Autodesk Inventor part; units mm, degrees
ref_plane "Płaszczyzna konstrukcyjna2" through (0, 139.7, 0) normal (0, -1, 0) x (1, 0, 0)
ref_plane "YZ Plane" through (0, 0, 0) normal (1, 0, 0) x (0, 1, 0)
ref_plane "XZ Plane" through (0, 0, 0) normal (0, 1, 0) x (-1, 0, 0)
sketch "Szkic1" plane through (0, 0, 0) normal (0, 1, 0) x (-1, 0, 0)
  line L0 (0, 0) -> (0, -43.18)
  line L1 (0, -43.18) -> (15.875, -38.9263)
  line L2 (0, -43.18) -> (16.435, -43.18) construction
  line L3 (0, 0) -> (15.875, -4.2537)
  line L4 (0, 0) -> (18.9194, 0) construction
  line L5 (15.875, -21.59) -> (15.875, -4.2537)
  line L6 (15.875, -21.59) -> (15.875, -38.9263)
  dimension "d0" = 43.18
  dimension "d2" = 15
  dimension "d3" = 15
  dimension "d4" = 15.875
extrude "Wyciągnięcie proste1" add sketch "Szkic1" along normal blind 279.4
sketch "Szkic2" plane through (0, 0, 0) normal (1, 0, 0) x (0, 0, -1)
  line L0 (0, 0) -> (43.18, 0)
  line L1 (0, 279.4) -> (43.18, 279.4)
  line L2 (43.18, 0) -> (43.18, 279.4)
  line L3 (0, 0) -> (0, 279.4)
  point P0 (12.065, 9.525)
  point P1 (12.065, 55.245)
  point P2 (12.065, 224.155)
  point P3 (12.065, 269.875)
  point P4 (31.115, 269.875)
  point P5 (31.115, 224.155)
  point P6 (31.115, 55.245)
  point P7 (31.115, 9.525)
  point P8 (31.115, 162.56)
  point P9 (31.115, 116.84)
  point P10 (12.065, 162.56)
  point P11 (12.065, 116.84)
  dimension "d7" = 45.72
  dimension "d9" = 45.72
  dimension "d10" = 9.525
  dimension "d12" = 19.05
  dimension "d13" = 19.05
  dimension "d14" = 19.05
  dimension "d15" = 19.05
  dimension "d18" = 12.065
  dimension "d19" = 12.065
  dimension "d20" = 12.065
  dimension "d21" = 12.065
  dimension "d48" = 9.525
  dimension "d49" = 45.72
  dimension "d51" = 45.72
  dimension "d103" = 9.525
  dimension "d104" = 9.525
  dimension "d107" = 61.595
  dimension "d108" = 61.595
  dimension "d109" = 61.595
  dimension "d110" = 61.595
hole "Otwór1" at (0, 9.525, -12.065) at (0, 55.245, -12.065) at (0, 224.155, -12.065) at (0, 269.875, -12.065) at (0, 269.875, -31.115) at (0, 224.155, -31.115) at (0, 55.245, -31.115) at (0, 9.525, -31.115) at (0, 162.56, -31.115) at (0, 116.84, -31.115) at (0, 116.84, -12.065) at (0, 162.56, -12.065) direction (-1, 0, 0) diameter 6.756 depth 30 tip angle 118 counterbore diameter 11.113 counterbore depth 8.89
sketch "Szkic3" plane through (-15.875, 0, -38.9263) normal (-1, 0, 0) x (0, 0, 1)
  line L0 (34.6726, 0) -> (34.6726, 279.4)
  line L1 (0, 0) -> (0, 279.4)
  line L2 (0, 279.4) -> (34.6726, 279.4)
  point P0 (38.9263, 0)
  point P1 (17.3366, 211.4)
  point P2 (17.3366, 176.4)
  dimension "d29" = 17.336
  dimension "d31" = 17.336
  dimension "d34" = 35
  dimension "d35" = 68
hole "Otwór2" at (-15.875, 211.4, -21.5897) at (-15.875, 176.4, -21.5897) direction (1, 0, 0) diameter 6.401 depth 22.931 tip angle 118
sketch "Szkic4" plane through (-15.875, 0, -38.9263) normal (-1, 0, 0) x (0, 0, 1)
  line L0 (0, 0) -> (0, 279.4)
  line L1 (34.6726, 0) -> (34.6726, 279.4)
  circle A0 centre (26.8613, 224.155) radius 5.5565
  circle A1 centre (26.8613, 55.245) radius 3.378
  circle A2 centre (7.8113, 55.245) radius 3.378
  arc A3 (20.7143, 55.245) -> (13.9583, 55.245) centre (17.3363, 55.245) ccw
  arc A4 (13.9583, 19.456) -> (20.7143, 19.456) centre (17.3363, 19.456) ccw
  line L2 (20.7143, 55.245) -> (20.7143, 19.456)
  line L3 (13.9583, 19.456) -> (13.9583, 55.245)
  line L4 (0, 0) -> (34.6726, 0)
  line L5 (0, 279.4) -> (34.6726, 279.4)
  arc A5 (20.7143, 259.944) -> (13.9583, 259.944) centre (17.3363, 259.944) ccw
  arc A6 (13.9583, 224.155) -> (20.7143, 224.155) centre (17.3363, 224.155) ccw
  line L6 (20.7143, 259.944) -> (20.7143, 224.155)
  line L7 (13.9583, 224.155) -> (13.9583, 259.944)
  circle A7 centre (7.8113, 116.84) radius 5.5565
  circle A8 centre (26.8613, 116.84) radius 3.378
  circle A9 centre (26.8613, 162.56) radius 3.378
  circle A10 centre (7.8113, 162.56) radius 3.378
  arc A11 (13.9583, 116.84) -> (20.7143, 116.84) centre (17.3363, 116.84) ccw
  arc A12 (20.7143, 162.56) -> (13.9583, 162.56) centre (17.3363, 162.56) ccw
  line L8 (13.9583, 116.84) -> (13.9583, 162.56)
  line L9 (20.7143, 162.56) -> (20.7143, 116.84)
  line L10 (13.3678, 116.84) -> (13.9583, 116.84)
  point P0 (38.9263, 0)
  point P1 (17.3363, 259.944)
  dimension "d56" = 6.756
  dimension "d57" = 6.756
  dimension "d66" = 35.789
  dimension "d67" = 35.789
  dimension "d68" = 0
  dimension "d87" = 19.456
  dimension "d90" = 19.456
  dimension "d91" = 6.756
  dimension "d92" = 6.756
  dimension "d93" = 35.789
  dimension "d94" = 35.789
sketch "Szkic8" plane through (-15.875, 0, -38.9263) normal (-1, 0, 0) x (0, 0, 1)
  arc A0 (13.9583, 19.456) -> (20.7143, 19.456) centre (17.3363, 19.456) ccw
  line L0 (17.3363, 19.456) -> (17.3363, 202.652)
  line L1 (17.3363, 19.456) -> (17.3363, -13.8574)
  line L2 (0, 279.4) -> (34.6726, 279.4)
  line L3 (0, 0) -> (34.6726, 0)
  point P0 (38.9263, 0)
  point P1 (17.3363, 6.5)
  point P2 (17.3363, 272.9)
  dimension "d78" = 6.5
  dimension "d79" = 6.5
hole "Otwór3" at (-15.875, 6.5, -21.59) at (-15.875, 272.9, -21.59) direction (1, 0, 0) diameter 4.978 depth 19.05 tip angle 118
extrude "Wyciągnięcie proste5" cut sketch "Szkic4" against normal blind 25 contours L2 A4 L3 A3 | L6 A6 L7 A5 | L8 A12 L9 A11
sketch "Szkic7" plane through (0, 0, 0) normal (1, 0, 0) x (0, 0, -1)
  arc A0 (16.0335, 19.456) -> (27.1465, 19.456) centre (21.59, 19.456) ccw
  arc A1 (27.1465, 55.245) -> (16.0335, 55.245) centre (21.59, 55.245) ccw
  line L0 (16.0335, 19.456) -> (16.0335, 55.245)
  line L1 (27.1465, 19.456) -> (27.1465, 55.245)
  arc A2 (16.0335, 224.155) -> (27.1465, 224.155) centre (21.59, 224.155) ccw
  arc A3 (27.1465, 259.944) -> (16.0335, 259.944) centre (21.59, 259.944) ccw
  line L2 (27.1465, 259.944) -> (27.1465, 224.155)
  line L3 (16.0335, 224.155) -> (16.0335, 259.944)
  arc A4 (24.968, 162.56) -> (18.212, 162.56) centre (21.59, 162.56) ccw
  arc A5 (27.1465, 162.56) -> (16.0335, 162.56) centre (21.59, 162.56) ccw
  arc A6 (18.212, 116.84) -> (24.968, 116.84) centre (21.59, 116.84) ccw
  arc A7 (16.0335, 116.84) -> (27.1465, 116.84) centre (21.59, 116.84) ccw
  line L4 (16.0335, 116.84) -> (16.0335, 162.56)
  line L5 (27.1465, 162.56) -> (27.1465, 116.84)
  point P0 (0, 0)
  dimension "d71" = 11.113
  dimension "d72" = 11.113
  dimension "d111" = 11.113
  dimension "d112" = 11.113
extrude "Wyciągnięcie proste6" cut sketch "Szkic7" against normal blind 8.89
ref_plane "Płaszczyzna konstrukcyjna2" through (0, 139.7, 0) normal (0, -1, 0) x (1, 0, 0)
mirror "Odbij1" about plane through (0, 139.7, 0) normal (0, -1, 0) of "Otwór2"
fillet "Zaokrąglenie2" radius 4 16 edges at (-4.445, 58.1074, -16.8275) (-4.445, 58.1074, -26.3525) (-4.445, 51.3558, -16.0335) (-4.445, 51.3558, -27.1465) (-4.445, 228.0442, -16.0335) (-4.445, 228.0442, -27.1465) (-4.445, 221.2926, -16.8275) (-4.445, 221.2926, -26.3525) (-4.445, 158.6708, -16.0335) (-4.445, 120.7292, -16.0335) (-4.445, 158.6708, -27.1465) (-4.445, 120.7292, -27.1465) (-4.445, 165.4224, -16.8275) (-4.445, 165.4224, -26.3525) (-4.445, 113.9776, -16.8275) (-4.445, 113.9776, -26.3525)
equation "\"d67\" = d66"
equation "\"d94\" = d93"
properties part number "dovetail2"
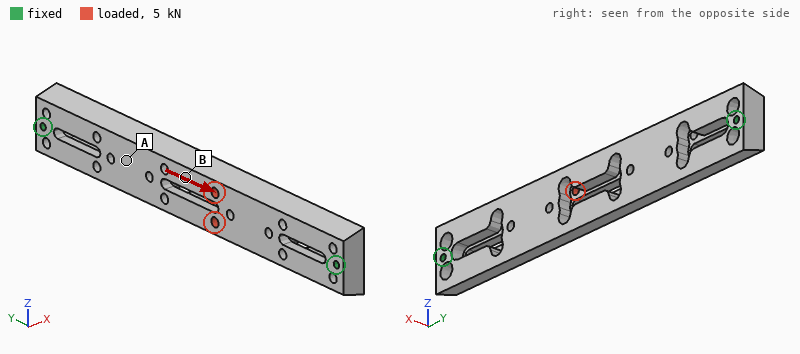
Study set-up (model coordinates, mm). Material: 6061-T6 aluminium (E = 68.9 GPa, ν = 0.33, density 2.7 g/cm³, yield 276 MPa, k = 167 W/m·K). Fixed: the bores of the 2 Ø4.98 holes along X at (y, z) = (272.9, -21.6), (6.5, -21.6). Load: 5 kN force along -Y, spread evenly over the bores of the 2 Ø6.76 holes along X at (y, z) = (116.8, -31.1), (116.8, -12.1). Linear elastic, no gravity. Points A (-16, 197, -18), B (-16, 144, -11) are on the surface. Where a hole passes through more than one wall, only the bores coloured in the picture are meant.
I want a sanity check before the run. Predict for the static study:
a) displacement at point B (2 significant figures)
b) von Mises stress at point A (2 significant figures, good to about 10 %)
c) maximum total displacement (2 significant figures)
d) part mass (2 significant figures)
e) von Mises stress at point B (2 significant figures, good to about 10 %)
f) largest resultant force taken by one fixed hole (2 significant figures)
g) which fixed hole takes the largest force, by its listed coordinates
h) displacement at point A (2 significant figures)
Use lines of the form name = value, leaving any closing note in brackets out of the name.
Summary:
displacement at point B = 30 µm
von Mises stress at point A = 5.2 MPa
maximum total displacement = 31 µm
part mass = 370 g
von Mises stress at point B = 12 MPa
largest resultant force taken by one fixed hole = 2.9 kN
which fixed hole takes the largest force, by its listed coordinates = (6.5, -21.6)
displacement at point A = 24 µm
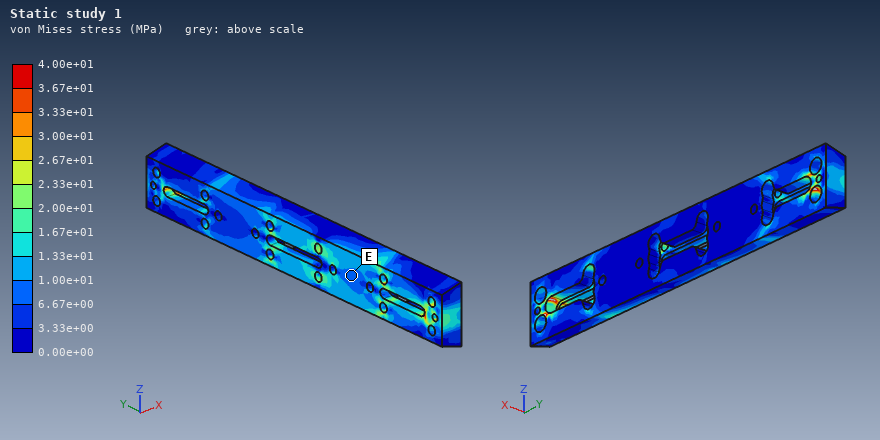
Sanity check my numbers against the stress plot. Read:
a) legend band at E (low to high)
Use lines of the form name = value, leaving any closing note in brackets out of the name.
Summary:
legend band at E = 6.67e+00 to 1.00e+01 MPa
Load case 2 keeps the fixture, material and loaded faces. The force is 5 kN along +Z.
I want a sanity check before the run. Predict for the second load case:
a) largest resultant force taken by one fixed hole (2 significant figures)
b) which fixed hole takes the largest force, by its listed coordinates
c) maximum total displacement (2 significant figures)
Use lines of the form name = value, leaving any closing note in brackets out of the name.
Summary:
largest resultant force taken by one fixed hole = 3.0 kN
which fixed hole takes the largest force, by its listed coordinates = (6.5, -21.6)
maximum total displacement = 0.42 mm
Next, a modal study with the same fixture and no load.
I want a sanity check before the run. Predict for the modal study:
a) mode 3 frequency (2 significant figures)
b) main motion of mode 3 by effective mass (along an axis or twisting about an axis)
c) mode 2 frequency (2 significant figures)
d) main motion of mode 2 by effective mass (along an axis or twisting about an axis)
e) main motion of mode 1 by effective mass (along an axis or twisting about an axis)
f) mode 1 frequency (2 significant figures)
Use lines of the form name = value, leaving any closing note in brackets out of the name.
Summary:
mode 3 frequency = 2400 Hz
main motion of mode 3 by effective mass = twisting about Z
mode 2 frequency = 1300 Hz
main motion of mode 2 by effective mass = along Z
main motion of mode 1 by effective mass = along X
mode 1 frequency = 870 Hz
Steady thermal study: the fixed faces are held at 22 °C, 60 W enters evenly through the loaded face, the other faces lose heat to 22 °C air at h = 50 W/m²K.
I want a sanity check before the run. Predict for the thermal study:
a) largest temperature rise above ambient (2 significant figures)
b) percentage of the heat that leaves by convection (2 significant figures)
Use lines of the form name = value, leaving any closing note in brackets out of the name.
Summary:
largest temperature rise above ambient = 41 K
percentage of the heat that leaves by convection = 51 %
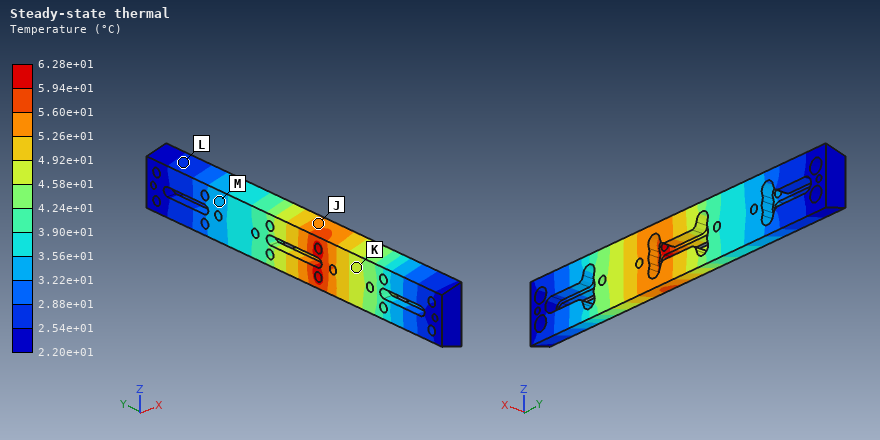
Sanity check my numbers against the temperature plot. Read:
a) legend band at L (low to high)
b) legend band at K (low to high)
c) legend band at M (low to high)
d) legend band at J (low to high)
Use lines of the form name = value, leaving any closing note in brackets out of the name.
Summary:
legend band at L = 2.54e+01 to 2.88e+01 °C
legend band at K = 4.58e+01 to 4.92e+01 °C
legend band at M = 3.22e+01 to 3.56e+01 °C
legend band at J = 5.26e+01 to 5.60e+01 °C
